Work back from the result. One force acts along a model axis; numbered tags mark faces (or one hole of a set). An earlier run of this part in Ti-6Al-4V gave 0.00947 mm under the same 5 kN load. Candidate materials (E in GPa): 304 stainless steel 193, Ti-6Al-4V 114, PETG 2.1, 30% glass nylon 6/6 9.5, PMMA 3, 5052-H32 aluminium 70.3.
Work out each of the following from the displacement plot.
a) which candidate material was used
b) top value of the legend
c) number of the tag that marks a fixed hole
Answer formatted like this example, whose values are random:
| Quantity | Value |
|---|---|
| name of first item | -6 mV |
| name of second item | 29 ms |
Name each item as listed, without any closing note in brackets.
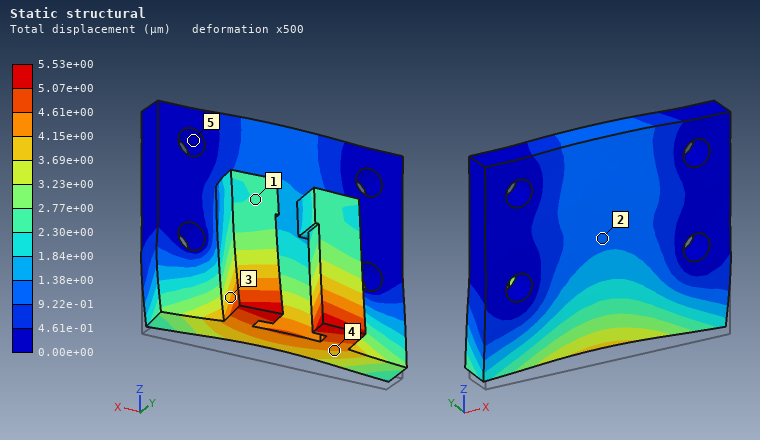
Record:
| Quantity | Value |
|---|---|
| which candidate material was used | 304 stainless steel |
| top value of the legend | 5.53e+00 µm |
| number of the tag that marks a fixed hole | 5 |
